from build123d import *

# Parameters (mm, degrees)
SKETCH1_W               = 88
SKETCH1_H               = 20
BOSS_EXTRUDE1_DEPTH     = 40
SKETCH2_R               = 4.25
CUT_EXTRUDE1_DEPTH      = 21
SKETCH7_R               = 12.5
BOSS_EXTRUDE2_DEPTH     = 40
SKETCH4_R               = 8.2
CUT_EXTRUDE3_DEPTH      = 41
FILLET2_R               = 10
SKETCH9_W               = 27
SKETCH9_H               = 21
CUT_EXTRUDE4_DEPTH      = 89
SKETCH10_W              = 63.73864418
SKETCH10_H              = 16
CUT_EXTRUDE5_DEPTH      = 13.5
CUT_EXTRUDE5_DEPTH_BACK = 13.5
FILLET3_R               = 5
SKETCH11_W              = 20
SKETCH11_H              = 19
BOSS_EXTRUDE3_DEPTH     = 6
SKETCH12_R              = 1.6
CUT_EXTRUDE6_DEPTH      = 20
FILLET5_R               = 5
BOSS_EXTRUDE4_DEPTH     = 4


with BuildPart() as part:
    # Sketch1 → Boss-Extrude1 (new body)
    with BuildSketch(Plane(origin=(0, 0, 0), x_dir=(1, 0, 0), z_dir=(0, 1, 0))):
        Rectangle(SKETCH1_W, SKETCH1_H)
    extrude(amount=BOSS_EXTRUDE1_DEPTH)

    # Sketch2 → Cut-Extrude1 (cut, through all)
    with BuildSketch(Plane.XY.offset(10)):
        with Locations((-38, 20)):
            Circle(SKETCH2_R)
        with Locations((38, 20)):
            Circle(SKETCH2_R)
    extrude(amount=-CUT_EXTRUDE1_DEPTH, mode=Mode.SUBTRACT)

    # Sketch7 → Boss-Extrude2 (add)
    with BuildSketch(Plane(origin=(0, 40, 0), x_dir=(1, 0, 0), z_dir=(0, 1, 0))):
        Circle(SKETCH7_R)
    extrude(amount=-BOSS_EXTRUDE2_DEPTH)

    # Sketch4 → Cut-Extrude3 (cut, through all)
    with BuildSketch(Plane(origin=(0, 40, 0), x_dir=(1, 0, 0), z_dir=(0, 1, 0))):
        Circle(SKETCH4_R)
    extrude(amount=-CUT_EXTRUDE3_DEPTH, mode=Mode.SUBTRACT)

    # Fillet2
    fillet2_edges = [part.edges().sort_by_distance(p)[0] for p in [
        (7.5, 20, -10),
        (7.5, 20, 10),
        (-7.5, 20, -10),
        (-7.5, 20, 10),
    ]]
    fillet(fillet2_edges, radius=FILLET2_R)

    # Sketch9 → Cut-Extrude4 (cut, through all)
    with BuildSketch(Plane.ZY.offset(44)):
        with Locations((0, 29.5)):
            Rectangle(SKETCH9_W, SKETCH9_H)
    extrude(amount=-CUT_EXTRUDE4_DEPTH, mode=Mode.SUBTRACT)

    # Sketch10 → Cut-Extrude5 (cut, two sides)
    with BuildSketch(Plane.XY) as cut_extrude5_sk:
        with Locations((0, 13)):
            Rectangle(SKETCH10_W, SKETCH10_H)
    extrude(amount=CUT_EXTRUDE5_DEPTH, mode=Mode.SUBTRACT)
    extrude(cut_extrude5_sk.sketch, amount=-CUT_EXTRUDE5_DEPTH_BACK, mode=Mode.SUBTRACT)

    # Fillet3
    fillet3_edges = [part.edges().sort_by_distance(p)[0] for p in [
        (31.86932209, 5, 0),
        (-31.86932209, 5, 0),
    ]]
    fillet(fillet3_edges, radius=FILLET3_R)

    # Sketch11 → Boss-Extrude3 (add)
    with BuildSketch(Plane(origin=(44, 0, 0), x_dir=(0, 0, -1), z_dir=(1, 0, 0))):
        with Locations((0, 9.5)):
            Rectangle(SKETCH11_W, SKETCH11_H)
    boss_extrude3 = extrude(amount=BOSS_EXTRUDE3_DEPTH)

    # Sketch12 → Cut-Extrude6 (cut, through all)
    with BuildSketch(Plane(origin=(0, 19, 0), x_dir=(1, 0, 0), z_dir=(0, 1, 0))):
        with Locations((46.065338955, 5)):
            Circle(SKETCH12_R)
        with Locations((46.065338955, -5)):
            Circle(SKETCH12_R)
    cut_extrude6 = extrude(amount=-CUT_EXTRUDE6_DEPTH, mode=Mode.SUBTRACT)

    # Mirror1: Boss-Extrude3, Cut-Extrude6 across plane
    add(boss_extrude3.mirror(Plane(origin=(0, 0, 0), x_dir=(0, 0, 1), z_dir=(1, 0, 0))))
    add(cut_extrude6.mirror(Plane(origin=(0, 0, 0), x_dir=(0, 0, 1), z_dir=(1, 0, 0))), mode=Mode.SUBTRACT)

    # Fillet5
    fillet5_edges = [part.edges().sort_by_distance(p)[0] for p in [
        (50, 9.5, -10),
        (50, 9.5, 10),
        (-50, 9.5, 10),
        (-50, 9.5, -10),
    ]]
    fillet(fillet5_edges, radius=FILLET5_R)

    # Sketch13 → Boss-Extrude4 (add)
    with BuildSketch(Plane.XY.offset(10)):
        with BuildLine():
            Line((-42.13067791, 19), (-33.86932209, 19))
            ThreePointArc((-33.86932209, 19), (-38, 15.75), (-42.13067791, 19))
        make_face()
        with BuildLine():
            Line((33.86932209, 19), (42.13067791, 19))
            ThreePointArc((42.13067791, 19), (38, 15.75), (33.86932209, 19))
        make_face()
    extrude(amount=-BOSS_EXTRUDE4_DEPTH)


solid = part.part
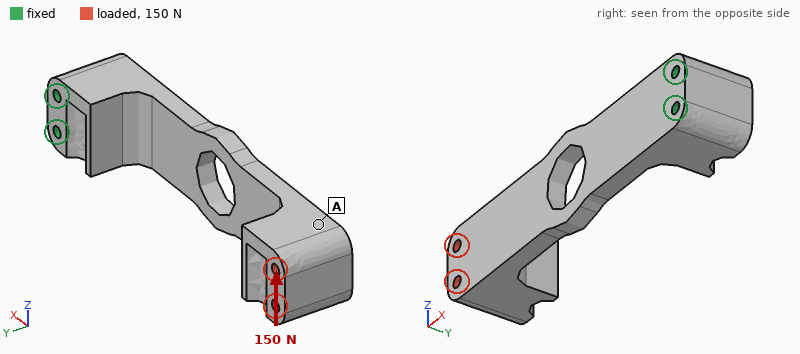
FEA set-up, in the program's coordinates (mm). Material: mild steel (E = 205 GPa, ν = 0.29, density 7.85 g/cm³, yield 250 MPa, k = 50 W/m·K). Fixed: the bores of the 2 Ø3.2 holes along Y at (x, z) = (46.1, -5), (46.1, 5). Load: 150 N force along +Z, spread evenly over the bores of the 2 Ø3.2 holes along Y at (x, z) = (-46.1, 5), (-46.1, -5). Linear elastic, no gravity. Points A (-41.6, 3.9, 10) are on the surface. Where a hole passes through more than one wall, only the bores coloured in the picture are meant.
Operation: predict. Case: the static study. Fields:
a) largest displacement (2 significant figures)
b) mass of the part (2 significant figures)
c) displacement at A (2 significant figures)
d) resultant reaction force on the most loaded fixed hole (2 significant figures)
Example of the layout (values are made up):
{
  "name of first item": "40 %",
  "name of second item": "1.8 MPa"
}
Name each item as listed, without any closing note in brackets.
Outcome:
{
  "largest displacement": "86 µm",
  "mass of the part": "140 g",
  "displacement at A": "58 µm",
  "resultant reaction force on the most loaded fixed hole": "1.1 kN"
}
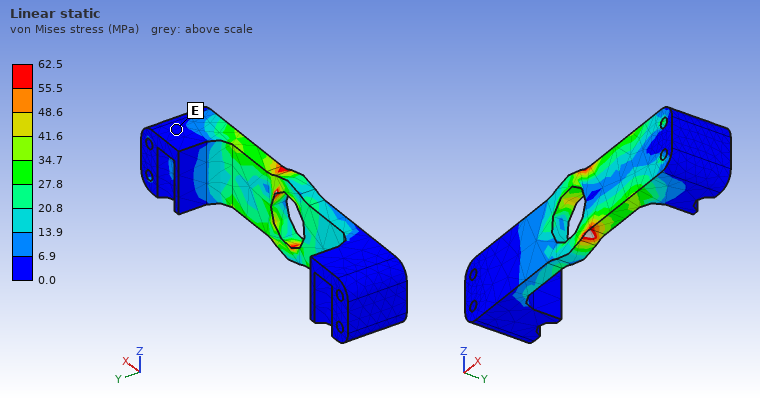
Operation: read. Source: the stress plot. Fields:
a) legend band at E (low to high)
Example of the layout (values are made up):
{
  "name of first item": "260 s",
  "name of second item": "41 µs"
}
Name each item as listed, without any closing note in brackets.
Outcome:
{
  "legend band at E": "0.0 to 6.9 MPa"
}
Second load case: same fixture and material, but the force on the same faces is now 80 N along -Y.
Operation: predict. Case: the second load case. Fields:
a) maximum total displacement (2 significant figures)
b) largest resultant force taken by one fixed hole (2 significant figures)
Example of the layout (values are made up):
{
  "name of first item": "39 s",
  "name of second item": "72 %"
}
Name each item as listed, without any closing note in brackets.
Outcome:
{
  "maximum total displacement": "0.46 mm",
  "largest resultant force taken by one fixed hole": "43 N"
}
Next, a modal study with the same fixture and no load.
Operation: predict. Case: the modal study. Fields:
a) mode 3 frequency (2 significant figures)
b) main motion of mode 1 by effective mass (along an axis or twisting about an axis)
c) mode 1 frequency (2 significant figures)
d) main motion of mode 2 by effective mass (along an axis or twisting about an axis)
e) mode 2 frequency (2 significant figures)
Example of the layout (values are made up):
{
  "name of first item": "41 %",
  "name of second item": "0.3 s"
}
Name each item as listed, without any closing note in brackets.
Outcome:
{
  "mode 3 frequency": "2400 Hz",
  "main motion of mode 1 by effective mass": "along Y",
  "mode 1 frequency": "330 Hz",
  "main motion of mode 2 by effective mass": "along Z",
  "mode 2 frequency": "1100 Hz"
}
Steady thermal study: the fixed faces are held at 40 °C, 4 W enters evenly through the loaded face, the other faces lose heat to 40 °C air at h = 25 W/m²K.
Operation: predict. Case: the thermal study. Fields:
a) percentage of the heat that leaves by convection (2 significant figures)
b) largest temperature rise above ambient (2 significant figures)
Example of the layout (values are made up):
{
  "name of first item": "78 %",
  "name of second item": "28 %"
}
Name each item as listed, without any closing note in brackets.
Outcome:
{
  "percentage of the heat that leaves by convection": "68 %",
  "largest temperature rise above ambient": "34 K"
}
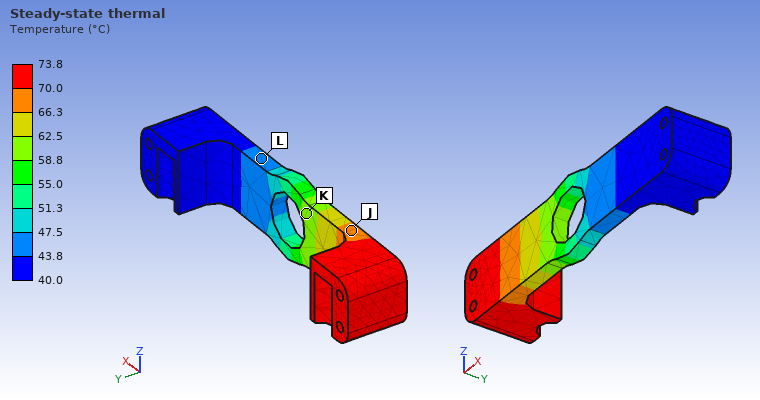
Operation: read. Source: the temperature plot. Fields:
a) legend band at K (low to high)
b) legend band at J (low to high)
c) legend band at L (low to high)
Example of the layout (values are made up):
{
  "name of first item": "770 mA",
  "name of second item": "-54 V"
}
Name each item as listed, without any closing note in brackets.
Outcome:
{
  "legend band at K": "58.8 to 62.5 °C",
  "legend band at J": "66.3 to 70.0 °C",
  "legend band at L": "43.8 to 47.5 °C"
}
